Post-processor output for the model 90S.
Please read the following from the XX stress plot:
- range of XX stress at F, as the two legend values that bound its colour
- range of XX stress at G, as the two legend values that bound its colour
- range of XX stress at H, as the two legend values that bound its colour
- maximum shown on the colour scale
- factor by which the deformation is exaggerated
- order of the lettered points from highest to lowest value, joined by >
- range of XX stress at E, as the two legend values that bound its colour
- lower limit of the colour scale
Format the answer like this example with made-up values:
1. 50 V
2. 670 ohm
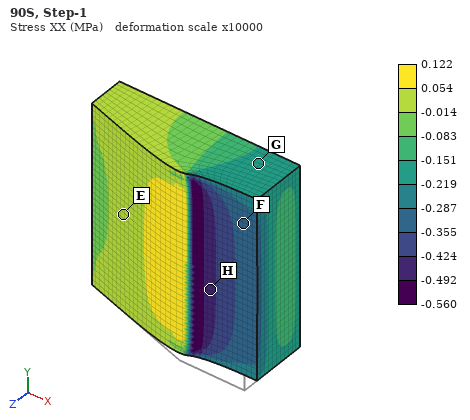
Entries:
1. -0.355 to -0.287 MPa
2. -0.219 to -0.151 MPa
3. -0.492 to -0.424 MPa
4. 0.122 MPa
5. 10000
6. E > G > F > H
7. -0.014 to 0.054 MPa
8. -0.560 MPa
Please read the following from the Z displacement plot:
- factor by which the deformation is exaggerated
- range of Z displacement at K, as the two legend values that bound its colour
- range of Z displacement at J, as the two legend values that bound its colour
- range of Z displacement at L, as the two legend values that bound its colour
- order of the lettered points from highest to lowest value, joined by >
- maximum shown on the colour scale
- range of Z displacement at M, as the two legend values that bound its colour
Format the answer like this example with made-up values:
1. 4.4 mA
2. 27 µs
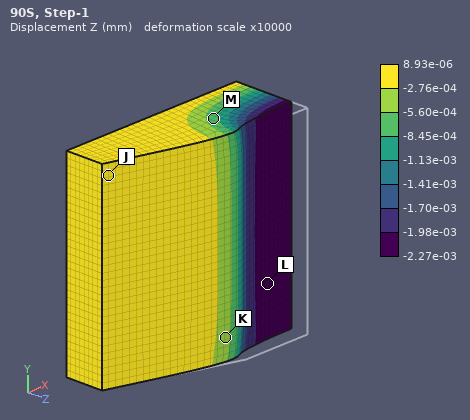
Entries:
1. 10000
2. -5.60e-04 to -2.76e-04 mm
3. -2.76e-04 to 8.93e-06 mm
4. -2.27e-03 to -1.98e-03 mm
5. J > K > M > L
6. 8.93e-06 mm
7. -8.45e-04 to -5.60e-04 mm
